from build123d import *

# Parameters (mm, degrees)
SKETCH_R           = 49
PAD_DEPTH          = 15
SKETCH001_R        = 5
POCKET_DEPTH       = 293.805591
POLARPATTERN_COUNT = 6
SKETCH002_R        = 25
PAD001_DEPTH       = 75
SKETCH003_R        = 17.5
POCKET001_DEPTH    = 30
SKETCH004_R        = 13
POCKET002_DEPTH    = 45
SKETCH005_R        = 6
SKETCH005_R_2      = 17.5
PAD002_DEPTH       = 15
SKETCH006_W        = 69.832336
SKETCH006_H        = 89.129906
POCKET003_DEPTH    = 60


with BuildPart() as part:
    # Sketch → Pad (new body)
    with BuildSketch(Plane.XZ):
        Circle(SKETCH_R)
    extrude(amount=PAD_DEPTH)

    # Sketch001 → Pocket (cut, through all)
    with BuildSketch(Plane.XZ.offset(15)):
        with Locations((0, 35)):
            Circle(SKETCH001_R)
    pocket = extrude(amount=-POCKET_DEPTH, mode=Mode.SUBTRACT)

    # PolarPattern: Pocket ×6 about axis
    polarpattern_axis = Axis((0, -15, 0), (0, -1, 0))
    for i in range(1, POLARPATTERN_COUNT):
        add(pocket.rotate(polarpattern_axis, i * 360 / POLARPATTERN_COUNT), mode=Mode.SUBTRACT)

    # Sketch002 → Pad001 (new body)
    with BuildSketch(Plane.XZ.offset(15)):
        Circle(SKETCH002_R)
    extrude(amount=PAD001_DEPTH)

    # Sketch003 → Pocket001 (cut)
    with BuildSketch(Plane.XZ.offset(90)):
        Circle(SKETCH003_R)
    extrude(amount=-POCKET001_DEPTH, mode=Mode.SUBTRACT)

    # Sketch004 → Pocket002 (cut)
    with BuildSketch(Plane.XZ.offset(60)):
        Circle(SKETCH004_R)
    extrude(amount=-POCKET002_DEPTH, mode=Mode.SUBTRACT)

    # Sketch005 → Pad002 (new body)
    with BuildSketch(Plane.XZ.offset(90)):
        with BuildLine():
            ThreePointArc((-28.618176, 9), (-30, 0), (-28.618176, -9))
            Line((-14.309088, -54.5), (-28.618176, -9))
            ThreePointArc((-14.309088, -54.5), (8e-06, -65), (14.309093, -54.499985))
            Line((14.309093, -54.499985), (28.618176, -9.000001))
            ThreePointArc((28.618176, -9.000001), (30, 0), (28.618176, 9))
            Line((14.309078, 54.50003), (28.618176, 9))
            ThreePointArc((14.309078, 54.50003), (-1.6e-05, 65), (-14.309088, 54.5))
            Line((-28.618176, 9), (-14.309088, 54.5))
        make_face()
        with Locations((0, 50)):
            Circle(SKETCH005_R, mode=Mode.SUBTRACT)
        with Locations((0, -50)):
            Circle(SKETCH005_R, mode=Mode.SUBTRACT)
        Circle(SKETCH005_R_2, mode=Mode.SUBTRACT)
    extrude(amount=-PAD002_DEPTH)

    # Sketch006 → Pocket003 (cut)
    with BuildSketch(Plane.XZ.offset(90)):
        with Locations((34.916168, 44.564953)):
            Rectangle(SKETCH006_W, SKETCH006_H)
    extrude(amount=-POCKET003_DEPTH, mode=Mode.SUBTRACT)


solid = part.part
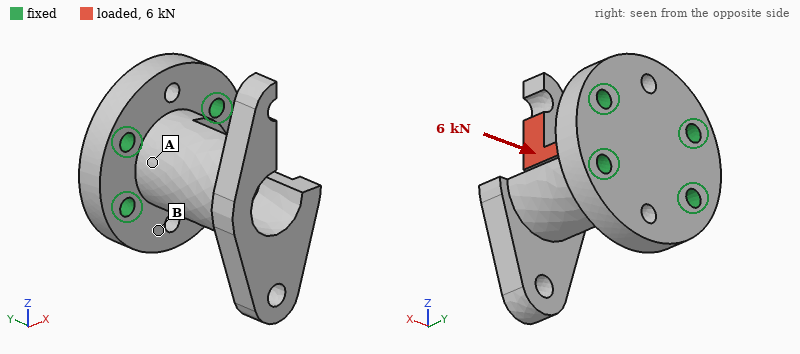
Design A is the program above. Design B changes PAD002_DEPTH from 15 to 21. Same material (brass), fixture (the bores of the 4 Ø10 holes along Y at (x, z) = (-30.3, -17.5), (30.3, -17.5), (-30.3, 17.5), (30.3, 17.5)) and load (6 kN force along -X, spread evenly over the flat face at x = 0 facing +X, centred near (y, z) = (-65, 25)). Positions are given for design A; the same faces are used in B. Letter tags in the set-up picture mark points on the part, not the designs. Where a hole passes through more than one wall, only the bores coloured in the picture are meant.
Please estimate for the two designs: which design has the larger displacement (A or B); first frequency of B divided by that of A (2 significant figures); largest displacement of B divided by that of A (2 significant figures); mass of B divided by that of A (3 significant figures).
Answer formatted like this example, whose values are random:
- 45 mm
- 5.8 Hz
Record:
- A
- 0.95
- 0.91
- 1.07
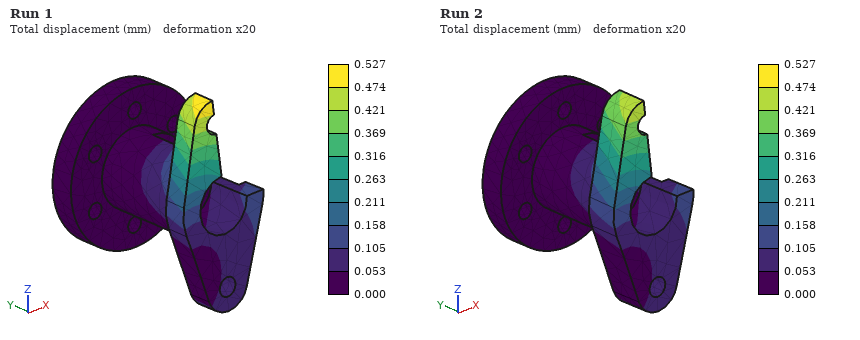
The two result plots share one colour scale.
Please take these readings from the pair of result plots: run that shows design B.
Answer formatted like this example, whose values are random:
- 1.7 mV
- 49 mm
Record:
- Run 2
